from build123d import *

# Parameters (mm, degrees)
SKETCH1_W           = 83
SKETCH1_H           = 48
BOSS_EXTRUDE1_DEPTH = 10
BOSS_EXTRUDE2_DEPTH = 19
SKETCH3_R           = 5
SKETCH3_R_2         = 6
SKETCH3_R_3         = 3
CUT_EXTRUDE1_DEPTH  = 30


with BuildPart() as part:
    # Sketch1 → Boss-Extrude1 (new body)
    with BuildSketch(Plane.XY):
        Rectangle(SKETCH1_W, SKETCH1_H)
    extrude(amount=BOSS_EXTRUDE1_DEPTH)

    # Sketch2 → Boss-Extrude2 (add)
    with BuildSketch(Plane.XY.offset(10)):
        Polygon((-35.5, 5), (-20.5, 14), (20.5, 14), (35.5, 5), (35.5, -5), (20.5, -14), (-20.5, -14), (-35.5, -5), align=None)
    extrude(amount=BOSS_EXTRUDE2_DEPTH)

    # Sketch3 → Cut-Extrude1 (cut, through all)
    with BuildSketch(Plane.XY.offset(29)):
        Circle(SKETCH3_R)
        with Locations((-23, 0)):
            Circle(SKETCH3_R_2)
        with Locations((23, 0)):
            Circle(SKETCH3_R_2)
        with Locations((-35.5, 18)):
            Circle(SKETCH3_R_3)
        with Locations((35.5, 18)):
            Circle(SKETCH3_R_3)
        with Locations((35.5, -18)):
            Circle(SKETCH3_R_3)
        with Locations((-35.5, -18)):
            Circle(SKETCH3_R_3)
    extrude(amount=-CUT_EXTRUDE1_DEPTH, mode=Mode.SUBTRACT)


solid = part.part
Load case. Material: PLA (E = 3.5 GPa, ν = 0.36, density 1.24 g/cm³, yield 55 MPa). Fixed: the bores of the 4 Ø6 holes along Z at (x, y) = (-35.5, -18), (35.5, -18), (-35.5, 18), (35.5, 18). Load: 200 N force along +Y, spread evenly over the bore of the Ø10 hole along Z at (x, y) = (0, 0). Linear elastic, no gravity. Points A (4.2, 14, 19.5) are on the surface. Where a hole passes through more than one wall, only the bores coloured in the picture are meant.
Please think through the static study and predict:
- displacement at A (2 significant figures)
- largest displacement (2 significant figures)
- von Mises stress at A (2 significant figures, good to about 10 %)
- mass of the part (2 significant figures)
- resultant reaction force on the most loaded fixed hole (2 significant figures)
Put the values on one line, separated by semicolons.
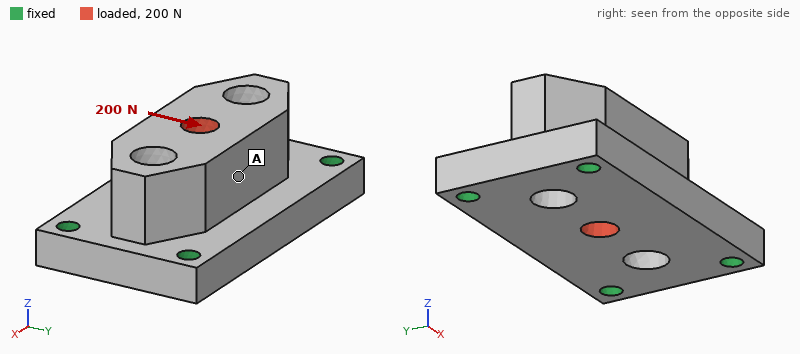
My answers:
10 µm; 13 µm; 0.30 MPa; 78 g; 71 N
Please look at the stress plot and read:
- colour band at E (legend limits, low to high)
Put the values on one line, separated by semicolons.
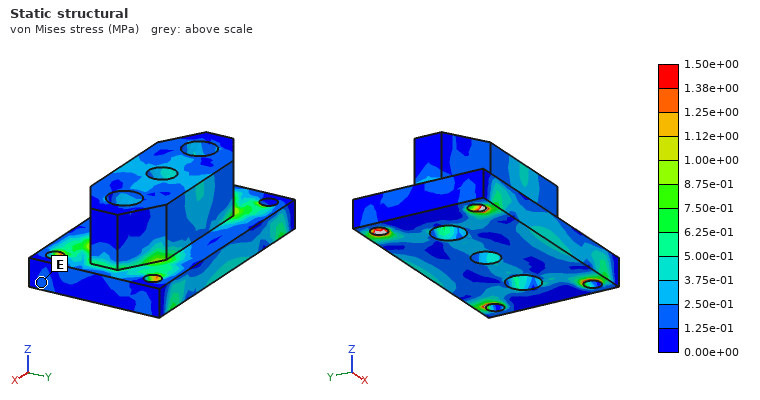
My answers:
1.25e-01 to 2.50e-01 MPa
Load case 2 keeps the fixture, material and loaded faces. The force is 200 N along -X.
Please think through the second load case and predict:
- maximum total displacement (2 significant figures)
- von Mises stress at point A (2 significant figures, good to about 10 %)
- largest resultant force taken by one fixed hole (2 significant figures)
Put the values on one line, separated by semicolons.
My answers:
4.4 µm; 0.11 MPa; 54 N
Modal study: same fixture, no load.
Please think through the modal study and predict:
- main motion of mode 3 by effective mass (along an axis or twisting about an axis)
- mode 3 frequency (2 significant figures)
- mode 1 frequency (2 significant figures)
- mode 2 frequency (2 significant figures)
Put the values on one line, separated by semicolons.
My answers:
along Y; 4800 Hz; 3100 Hz; 3200 Hz
